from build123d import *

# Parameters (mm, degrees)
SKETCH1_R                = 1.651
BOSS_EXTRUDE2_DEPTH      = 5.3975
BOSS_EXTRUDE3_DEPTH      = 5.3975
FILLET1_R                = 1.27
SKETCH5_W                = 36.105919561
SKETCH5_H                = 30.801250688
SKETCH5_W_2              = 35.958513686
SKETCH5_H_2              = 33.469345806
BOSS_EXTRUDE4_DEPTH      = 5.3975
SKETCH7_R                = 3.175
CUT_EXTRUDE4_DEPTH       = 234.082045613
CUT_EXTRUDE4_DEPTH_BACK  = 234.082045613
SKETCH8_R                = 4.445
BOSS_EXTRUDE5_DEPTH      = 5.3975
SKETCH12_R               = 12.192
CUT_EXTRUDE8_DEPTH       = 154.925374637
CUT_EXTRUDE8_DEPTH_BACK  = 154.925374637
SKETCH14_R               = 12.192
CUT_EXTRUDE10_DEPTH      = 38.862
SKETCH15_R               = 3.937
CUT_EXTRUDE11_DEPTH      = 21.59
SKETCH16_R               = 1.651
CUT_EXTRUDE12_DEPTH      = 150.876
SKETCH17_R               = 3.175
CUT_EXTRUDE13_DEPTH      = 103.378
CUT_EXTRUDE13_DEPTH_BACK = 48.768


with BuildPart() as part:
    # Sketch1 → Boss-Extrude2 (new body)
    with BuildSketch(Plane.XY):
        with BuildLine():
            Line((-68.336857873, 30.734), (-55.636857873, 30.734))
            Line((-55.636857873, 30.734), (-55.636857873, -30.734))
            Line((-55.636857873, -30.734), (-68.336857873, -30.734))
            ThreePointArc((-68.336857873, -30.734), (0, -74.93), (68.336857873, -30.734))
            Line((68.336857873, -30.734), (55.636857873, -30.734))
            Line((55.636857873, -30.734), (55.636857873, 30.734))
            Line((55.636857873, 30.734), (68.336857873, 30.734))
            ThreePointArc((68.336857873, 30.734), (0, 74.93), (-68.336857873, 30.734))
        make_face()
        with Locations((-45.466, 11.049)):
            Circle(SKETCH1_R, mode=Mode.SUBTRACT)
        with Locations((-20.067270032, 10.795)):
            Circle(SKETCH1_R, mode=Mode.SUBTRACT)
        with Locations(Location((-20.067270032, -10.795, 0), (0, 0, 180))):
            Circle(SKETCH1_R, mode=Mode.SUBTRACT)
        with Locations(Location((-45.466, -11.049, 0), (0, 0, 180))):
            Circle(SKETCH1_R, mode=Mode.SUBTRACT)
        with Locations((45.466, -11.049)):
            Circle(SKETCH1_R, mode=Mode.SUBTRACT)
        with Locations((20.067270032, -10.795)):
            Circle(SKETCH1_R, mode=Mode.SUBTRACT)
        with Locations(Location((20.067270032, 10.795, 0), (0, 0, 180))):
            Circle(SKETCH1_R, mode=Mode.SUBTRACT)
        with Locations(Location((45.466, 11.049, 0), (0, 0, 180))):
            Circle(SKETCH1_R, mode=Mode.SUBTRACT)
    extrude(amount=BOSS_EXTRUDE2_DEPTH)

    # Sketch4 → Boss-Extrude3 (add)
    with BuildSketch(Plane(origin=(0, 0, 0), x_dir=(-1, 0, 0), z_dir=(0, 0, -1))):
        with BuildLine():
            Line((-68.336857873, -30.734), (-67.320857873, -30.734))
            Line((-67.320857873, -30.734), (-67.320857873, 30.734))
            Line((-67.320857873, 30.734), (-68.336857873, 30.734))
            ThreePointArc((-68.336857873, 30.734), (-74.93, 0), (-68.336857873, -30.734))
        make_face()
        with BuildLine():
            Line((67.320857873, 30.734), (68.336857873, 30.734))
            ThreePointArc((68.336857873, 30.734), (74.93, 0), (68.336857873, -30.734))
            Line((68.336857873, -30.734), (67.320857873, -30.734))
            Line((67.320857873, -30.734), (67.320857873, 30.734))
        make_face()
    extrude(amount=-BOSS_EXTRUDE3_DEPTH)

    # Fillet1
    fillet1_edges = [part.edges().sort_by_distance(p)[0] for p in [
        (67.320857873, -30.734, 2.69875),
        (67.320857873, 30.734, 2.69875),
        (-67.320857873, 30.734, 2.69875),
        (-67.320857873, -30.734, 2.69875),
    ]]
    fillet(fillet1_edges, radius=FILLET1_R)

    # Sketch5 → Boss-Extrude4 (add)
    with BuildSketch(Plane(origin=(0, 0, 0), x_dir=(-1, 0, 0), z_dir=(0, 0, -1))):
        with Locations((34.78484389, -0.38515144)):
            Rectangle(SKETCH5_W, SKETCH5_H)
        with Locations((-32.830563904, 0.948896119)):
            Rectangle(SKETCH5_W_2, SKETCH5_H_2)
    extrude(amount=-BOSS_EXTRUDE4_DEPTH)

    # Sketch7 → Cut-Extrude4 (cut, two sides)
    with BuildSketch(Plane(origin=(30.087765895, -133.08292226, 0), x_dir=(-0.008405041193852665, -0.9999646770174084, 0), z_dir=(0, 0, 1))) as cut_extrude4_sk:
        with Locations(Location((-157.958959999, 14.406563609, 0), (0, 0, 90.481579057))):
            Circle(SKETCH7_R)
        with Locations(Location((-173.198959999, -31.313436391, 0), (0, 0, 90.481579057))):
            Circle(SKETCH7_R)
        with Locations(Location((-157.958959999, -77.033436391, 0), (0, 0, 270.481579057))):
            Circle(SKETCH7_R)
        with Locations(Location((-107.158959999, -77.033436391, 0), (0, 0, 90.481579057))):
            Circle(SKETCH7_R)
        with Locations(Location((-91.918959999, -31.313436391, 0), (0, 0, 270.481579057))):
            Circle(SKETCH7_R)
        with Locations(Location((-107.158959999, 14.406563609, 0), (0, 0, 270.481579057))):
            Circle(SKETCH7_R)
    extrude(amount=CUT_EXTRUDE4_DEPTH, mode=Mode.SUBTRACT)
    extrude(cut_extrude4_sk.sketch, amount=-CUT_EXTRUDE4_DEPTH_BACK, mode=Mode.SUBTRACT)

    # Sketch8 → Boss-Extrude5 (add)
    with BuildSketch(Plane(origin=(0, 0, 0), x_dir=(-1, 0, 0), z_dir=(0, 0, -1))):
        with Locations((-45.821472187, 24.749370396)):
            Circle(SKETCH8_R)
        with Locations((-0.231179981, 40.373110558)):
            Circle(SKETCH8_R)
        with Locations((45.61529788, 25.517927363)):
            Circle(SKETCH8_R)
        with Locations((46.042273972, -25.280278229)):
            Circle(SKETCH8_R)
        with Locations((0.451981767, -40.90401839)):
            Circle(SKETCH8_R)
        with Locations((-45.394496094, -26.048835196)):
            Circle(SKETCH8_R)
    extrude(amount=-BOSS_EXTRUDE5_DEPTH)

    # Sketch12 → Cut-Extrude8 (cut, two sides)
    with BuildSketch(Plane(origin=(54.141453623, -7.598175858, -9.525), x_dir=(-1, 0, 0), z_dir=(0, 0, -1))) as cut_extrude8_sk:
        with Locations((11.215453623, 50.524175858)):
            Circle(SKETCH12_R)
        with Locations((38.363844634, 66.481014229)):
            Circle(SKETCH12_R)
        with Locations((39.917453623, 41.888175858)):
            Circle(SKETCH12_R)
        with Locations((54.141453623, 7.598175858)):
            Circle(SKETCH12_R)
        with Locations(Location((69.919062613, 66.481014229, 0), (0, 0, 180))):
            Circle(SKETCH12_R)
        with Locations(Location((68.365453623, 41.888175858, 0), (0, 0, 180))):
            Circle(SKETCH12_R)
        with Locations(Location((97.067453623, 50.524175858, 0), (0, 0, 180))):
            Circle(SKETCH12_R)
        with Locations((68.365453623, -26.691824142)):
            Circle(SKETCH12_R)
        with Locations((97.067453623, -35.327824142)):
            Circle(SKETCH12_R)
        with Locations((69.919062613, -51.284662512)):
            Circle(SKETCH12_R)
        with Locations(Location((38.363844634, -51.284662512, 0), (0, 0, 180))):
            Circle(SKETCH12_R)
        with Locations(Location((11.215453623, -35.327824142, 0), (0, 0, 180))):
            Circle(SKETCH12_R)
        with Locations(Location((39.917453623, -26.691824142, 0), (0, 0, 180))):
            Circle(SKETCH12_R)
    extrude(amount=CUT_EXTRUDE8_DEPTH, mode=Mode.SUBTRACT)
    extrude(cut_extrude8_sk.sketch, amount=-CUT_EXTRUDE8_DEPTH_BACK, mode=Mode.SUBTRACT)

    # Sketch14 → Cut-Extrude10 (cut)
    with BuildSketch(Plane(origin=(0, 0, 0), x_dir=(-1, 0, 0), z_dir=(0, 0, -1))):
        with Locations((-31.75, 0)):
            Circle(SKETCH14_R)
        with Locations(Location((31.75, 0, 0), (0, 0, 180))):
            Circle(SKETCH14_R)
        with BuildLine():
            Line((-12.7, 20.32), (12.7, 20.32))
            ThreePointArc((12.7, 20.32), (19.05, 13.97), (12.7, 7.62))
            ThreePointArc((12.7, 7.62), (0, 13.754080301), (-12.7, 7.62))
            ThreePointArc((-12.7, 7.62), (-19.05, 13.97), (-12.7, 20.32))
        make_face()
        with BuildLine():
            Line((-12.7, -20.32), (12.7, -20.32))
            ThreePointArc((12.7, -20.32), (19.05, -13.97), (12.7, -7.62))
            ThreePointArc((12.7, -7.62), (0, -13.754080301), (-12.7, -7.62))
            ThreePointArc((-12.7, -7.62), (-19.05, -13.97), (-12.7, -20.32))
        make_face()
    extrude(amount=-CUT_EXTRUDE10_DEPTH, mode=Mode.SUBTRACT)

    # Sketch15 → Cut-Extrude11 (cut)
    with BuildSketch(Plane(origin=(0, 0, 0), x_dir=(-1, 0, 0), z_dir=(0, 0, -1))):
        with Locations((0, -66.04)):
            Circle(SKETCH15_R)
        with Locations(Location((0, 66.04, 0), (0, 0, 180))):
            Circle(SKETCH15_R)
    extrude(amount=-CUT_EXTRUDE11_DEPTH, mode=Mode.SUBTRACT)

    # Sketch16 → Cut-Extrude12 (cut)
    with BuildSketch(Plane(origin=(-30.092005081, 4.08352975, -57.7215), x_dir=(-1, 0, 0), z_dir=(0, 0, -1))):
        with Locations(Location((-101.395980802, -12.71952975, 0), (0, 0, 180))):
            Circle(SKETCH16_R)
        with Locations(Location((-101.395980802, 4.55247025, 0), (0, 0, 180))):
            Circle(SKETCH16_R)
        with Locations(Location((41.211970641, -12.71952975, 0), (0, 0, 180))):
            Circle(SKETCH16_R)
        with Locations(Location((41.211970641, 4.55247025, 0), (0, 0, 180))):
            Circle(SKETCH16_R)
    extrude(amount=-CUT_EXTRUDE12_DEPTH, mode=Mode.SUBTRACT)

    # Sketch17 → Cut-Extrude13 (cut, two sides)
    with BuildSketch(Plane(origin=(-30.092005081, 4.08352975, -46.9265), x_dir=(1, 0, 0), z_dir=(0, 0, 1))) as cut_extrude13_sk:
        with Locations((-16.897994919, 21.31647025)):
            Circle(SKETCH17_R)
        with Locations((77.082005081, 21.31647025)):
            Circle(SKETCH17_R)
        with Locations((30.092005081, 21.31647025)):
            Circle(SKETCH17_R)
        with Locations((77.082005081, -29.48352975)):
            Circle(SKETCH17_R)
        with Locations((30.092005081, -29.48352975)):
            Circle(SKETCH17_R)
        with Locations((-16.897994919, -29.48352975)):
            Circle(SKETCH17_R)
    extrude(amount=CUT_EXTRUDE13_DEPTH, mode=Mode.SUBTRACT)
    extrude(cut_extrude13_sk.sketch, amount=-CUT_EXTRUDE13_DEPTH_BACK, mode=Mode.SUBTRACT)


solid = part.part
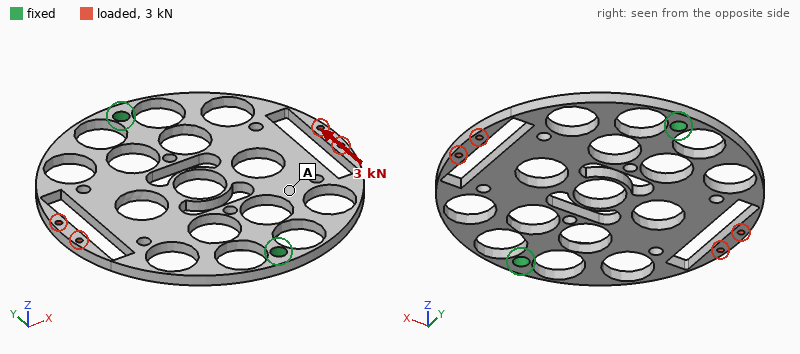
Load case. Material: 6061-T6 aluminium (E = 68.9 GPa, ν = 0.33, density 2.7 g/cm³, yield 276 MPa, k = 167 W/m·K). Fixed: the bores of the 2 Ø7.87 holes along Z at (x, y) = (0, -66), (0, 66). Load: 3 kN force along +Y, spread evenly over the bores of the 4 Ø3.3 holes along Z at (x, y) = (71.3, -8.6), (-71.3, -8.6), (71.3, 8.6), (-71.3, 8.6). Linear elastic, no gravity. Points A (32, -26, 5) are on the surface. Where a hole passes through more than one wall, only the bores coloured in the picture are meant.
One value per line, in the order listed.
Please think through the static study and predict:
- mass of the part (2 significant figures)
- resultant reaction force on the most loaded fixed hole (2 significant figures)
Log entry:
120 g
1.5 kN
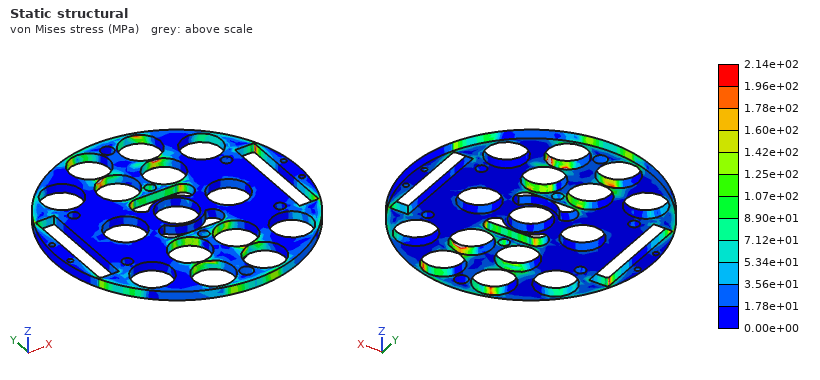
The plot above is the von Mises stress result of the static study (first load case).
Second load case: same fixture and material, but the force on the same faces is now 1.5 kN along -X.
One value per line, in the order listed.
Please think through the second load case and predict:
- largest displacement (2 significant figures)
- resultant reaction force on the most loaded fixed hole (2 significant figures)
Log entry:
0.28 mm
750 N
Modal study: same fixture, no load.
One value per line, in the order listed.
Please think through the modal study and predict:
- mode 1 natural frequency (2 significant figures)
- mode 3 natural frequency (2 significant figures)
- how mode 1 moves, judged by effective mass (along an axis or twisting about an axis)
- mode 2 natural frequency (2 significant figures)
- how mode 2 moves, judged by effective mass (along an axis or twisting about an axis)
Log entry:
370 Hz
1400 Hz
twisting about Y
490 Hz
along Z
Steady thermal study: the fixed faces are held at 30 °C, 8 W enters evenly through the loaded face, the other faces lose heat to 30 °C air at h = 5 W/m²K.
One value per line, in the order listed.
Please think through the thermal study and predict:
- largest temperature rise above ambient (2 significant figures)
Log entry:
33 K
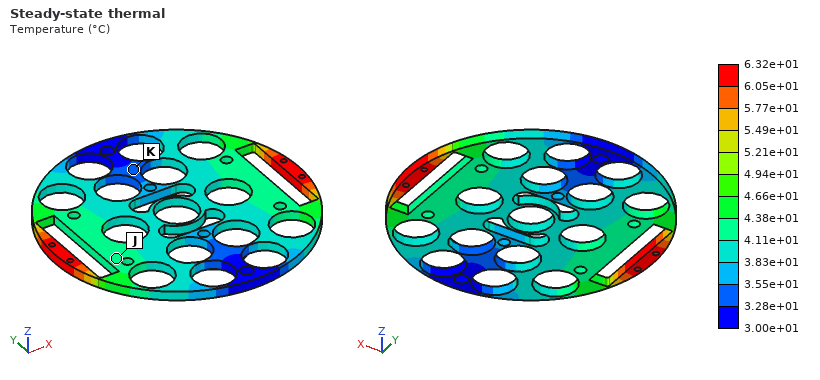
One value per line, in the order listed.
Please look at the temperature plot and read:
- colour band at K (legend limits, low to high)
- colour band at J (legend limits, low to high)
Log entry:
3.28e+01 to 3.55e+01 °C
4.11e+01 to 4.38e+01 °C
